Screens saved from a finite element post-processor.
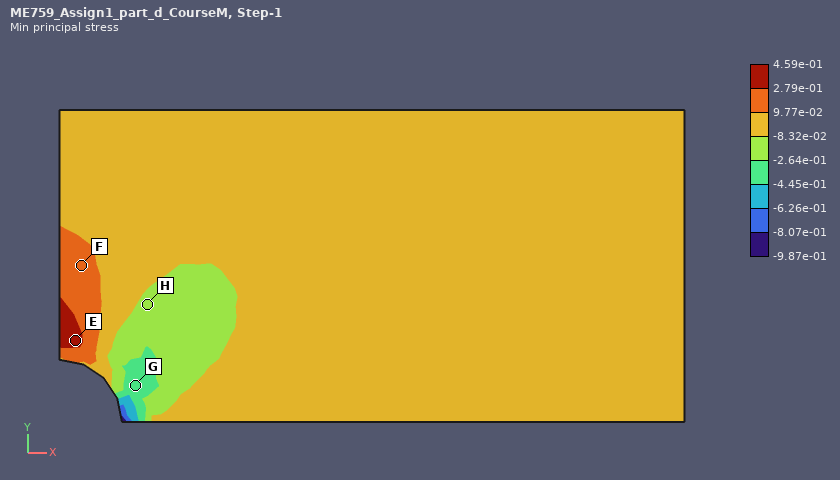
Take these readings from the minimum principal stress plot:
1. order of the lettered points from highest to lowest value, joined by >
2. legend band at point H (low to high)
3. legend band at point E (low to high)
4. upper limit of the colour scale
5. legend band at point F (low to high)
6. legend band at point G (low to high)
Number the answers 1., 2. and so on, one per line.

1. E > F > H > G
2. -2.64e-01 to -8.32e-02
3. 2.79e-01 to 4.59e-01
4. 4.59e-01
5. 9.77e-02 to 2.79e-01
6. -4.45e-01 to -2.64e-01
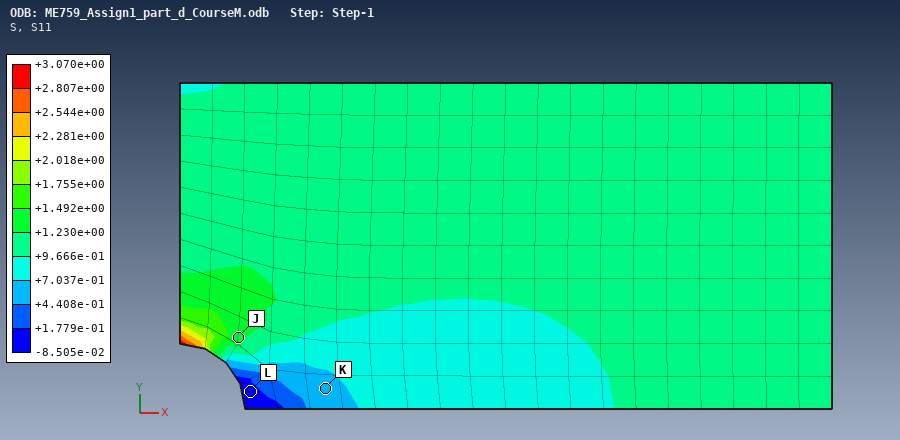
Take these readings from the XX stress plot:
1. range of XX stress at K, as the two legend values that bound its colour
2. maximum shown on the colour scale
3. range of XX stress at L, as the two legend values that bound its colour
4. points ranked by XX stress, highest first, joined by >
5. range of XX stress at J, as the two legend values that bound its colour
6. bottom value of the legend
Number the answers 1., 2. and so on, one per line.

1. +4.408e-01 to +7.037e-01
2. +3.070e+00
3. -8.505e-02 to +1.779e-01
4. J > K > L
5. +1.230e+00 to +1.492e+00
6. -8.505e-02
